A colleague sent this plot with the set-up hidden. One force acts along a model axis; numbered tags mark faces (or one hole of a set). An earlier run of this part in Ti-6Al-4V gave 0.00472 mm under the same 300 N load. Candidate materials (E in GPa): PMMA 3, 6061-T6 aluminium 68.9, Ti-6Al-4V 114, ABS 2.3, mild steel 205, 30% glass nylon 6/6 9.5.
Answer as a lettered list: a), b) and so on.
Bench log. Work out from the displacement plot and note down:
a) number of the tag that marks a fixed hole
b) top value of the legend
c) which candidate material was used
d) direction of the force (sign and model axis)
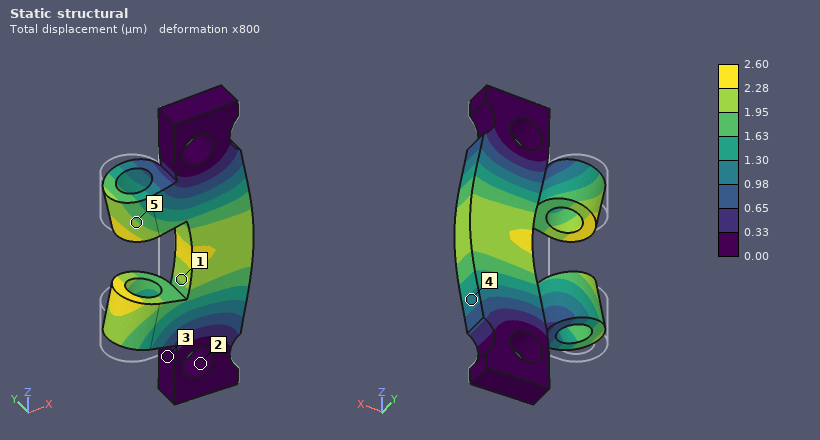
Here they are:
a) 2
b) 2.60 µm
c) mild steel
d) +X
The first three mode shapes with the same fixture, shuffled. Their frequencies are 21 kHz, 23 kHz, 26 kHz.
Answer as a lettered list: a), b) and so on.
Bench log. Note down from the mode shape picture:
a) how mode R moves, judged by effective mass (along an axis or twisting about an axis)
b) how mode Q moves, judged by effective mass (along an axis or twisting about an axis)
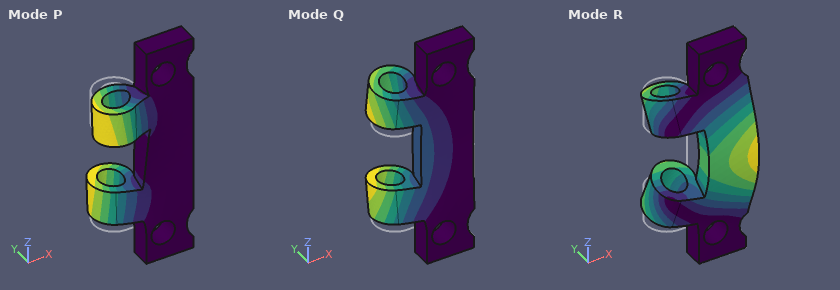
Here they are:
a) along Y
b) along Y
